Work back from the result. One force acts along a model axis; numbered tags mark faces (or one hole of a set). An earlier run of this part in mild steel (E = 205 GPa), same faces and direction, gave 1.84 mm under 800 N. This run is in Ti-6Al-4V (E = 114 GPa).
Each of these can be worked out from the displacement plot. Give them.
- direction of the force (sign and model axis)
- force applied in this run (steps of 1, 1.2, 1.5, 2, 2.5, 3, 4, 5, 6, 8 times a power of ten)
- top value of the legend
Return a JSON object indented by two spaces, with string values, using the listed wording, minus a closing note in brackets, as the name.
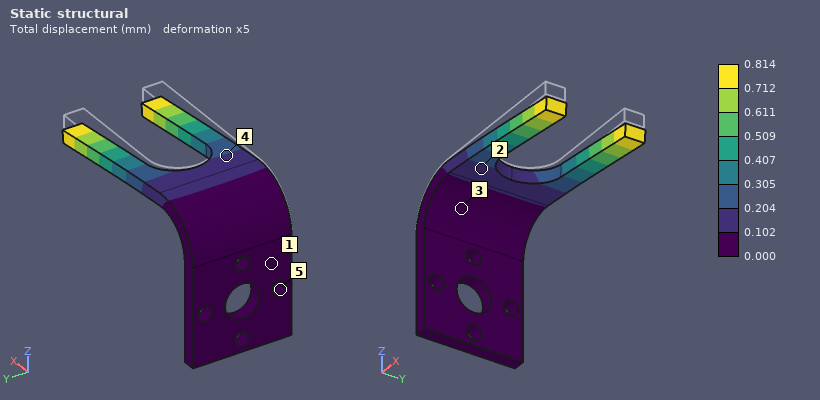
{
  "direction of the force": "-Z",
  "force applied in this run": "200 N",
  "top value of the legend": "0.814 mm"
}
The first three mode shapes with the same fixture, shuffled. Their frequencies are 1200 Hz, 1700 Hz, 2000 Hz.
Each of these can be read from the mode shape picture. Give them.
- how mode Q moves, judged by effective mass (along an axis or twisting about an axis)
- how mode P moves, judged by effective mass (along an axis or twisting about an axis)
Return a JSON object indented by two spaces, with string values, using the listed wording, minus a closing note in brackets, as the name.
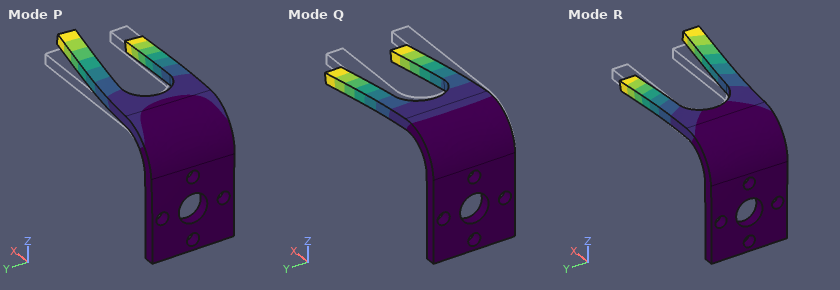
{
  "how mode Q moves, judged by effective mass": "along Z",
  "how mode P moves, judged by effective mass": "along Y"
}
